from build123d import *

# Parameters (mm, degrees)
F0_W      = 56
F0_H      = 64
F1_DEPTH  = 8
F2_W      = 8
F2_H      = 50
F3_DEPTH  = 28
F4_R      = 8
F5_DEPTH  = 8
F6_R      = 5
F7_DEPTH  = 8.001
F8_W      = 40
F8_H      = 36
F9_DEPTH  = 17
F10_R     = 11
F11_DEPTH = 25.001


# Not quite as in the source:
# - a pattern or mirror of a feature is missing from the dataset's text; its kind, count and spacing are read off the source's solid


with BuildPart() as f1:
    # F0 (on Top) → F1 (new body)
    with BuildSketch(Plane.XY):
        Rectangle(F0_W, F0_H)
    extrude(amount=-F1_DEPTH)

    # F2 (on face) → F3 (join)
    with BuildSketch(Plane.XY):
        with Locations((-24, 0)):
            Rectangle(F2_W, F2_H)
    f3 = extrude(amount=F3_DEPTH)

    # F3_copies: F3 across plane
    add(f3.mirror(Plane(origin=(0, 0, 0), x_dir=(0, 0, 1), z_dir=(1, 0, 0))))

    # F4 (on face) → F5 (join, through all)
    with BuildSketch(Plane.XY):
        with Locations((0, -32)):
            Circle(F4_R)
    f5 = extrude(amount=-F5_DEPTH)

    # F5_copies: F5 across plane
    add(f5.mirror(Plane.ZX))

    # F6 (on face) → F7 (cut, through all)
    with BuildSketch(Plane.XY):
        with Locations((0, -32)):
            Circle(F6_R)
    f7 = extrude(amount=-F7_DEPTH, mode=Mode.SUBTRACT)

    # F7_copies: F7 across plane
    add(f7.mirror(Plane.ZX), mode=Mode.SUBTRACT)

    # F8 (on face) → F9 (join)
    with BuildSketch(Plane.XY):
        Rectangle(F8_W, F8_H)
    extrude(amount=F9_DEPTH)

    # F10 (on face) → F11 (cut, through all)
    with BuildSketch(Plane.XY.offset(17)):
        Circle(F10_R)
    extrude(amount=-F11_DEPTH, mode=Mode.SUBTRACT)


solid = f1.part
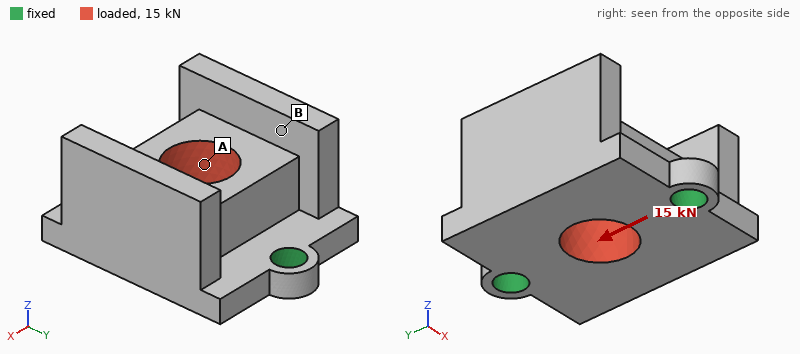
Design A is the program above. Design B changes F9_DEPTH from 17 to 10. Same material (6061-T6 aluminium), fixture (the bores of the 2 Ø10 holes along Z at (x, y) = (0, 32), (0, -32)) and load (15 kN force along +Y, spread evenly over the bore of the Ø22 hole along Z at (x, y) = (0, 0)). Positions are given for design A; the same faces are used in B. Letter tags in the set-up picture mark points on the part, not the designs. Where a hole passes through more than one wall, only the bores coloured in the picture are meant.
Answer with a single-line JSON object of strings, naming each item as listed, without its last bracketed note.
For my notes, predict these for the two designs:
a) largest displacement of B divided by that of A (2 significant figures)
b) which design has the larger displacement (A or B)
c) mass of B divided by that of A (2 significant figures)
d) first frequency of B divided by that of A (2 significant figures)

{"largest displacement of B divided by that of A": "0.66", "which design has the larger displacement": "A", "mass of B divided by that of A": "0.89", "first frequency of B divided by that of A": "1.0"}
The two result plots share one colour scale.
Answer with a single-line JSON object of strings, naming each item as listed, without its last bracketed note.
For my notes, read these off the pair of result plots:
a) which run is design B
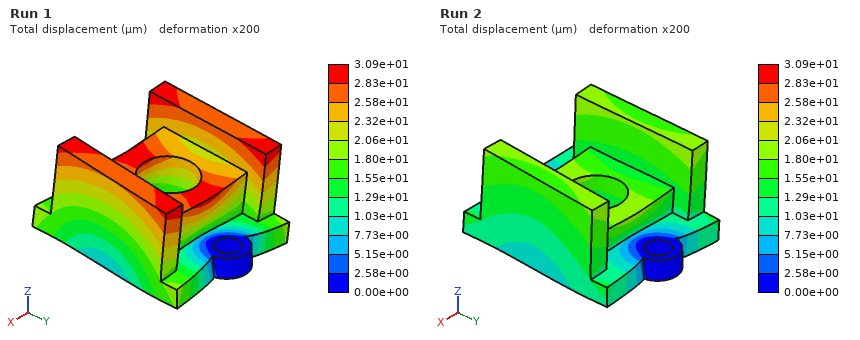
{"which run is design B": "Run 2"}
